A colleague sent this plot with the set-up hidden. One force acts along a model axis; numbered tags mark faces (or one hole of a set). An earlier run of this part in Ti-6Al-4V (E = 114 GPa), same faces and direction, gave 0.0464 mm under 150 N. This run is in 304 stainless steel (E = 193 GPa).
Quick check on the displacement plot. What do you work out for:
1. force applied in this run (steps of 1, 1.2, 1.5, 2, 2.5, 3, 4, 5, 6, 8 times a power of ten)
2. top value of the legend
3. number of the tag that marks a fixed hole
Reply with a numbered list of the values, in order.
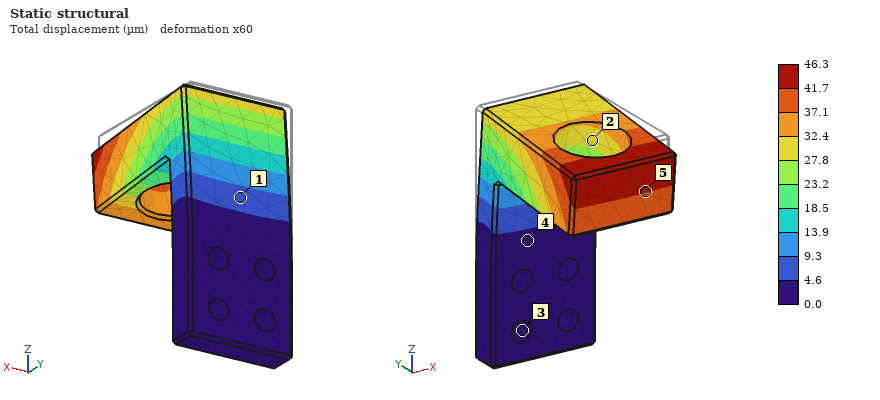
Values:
1. 250 N
2. 46.3 µm
3. 3
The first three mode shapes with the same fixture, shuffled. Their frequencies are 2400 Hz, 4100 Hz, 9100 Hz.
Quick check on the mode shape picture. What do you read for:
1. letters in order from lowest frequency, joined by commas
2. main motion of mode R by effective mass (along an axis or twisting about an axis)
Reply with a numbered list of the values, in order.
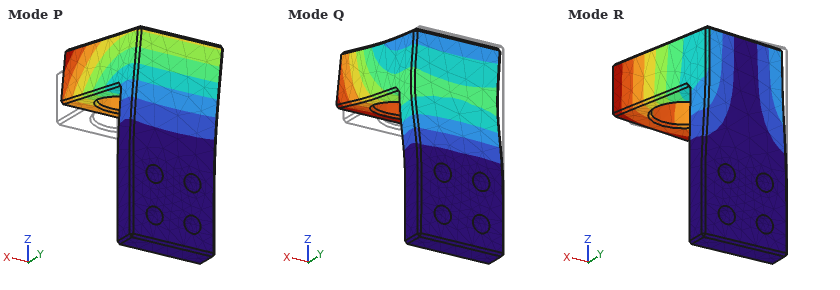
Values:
1. P, R, Q
2. along X
